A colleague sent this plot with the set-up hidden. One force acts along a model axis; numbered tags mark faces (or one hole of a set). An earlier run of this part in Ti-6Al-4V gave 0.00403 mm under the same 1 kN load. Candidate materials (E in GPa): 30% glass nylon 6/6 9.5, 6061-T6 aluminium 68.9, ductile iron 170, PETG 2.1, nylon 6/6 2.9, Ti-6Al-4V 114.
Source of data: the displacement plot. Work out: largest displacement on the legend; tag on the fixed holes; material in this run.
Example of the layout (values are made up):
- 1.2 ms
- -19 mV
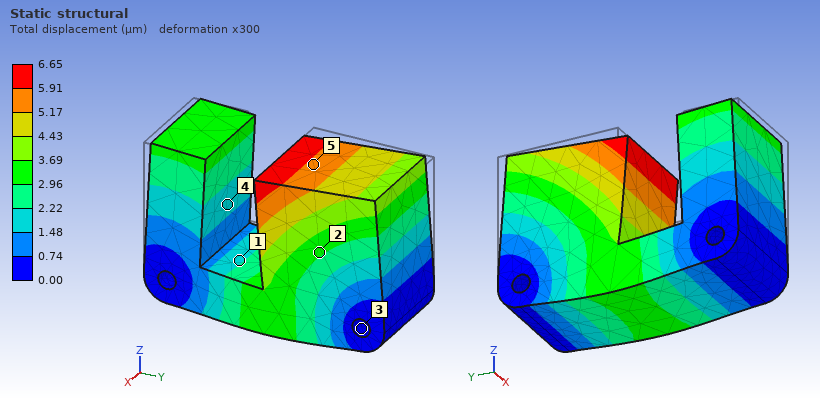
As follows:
- 6.65 µm
- 3
- 6061-T6 aluminium
